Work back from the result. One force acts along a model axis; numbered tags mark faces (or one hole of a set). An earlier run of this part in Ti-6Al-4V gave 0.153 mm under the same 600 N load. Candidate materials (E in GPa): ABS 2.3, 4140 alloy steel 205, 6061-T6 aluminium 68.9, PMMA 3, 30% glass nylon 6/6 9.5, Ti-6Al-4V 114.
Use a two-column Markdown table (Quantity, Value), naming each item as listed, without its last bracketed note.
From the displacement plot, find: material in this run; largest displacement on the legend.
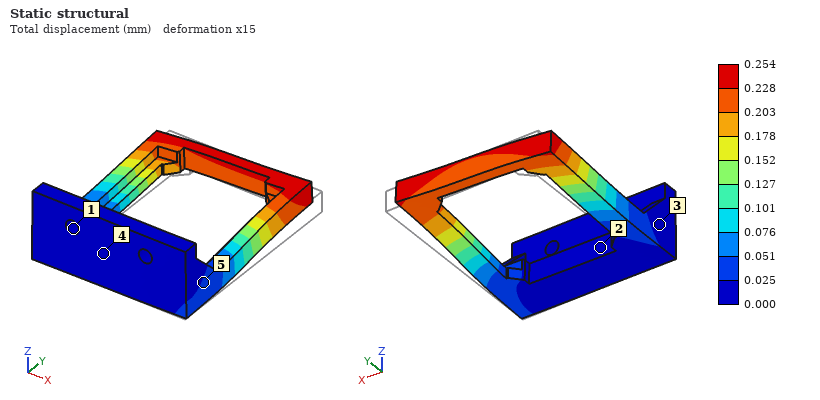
| Quantity | Value |
|---|---|
| material in this run | 6061-T6 aluminium |
| largest displacement on the legend | 0.254 mm |
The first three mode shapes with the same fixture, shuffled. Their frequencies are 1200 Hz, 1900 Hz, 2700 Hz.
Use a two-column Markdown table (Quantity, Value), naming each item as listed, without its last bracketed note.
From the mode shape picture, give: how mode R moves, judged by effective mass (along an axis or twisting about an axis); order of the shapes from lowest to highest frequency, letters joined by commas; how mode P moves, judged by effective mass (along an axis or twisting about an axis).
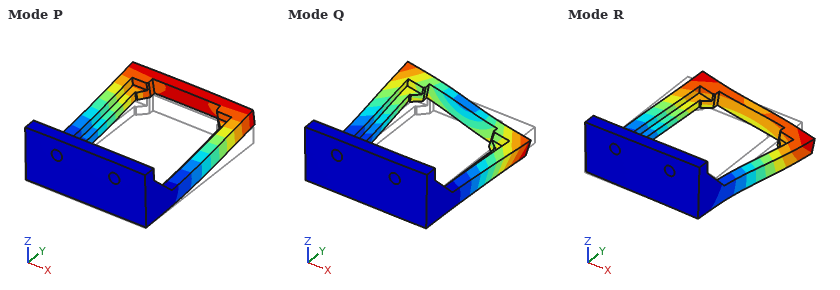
| Quantity | Value |
|---|---|
| how mode R moves, judged by effective mass | along X |
| order of the shapes from lowest to highest frequency, letters joined by commas | P, R, Q |
| how mode P moves, judged by effective mass | along Z |
